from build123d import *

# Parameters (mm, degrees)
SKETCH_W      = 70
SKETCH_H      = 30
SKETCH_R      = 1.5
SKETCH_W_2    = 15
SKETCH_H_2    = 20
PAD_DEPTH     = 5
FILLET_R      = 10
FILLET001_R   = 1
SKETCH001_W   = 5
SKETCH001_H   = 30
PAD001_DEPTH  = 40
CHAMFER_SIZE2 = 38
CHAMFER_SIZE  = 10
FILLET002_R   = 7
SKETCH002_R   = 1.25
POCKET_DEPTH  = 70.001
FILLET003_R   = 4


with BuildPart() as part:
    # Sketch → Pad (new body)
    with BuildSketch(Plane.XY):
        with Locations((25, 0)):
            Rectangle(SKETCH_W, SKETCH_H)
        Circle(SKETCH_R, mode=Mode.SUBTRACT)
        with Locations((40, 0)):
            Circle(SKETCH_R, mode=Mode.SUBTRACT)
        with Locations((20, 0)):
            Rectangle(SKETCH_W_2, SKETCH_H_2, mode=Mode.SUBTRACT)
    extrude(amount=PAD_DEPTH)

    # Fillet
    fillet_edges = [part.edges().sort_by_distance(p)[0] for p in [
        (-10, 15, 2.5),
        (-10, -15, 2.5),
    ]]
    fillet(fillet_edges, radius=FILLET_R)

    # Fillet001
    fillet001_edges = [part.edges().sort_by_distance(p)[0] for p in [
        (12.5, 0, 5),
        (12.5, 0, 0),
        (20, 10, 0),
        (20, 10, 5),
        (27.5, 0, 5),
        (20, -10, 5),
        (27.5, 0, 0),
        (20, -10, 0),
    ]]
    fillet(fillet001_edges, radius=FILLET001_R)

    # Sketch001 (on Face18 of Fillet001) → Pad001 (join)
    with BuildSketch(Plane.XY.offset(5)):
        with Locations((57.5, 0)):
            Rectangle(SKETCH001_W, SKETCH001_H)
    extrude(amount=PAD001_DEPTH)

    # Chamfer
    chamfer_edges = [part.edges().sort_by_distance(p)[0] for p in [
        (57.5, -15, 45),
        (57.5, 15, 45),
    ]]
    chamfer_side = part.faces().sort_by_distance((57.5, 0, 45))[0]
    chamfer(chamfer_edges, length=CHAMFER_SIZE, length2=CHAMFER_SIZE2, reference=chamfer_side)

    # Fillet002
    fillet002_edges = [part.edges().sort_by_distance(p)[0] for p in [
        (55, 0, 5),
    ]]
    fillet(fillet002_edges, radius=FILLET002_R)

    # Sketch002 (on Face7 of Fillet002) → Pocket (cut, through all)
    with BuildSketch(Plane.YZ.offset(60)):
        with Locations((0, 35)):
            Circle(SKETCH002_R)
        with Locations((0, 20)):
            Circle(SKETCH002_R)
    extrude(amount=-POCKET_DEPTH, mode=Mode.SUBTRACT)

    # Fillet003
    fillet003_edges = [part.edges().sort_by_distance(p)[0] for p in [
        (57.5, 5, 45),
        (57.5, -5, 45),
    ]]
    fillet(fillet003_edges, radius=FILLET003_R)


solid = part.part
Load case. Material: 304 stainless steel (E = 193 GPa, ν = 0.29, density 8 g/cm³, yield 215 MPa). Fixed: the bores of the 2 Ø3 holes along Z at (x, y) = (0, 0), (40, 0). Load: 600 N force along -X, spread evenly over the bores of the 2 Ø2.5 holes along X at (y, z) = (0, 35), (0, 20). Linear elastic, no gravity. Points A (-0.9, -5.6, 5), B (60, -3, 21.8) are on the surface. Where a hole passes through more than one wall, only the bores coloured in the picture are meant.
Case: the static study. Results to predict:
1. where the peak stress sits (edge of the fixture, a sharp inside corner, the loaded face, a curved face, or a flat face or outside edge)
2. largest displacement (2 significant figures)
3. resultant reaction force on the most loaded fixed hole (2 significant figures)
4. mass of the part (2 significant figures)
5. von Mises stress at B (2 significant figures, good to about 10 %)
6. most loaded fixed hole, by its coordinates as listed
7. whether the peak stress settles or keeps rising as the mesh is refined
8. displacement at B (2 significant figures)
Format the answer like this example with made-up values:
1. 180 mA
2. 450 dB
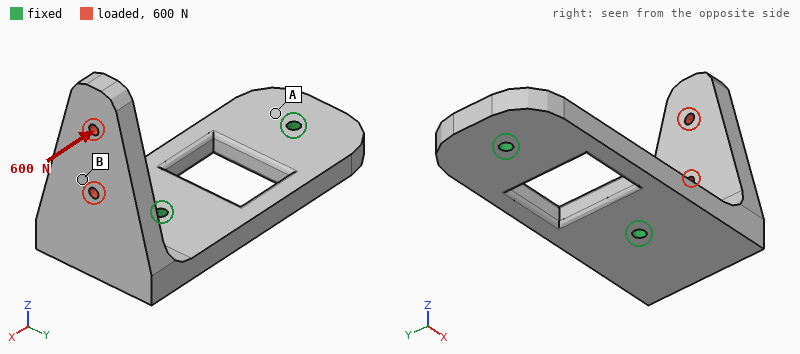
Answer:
1. edge of the fixture
2. 0.26 mm
3. 550 N
4. 100 g
5. 45 MPa
6. (40, 0)
7. keeps rising
8. 0.11 mm
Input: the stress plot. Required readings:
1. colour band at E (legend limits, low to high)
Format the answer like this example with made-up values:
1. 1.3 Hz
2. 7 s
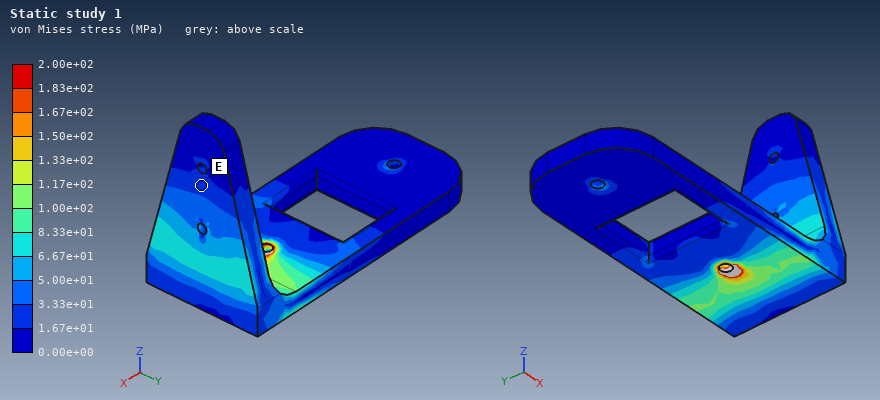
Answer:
1. 1.67e+01 to 3.33e+01 MPa
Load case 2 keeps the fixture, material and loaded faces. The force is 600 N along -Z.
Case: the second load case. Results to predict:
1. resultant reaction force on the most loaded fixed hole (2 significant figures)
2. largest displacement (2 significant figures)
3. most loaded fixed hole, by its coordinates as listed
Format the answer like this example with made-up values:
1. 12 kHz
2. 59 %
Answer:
1. 670 N
2. 85 µm
3. (40, 0)
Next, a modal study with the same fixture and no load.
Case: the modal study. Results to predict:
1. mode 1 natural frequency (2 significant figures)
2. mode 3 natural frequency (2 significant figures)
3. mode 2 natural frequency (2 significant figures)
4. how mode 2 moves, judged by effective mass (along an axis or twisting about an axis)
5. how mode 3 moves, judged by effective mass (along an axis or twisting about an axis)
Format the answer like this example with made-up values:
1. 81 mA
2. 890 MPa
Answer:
1. 1900 Hz
2. 5800 Hz
3. 2700 Hz
4. along Y
5. along Z
